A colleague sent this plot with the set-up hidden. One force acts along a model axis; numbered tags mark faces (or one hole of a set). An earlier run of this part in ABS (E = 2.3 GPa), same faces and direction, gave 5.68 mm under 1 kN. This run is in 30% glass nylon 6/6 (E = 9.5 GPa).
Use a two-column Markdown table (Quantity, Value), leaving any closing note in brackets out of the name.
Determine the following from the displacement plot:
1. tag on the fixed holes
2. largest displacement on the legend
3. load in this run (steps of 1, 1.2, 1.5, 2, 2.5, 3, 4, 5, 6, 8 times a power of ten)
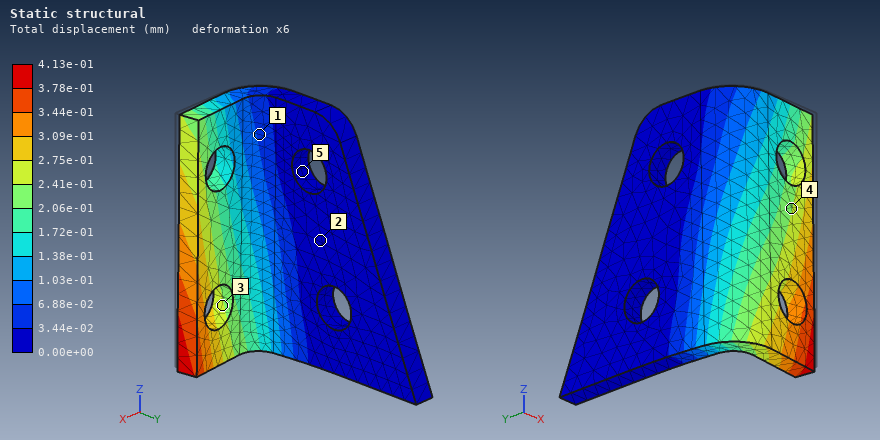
| Quantity | Value |
|---|---|
| tag on the fixed holes | 5 |
| largest displacement on the legend | 4.13e-01 mm |
| load in this run | 300 N |
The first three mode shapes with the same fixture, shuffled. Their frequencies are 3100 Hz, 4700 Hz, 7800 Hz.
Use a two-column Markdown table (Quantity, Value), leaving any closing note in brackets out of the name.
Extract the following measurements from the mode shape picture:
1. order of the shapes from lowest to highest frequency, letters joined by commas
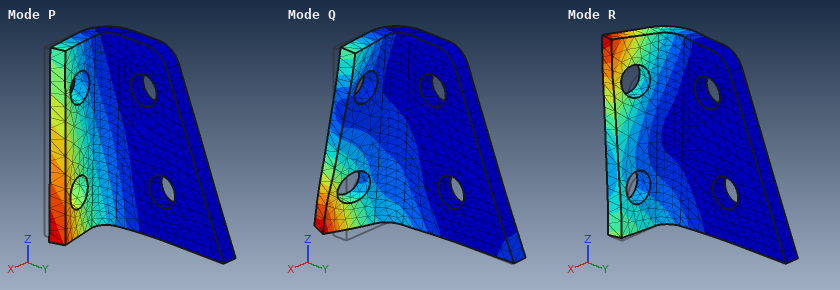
| Quantity | Value |
|---|---|
| order of the shapes from lowest to highest frequency, letters joined by commas | P, R, Q |
